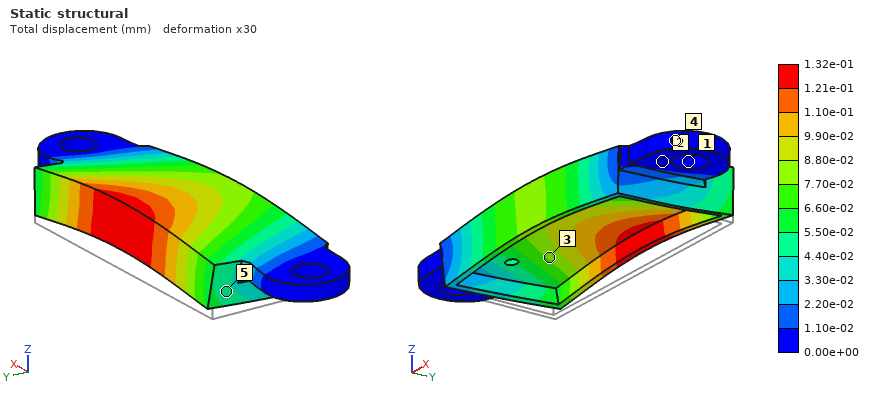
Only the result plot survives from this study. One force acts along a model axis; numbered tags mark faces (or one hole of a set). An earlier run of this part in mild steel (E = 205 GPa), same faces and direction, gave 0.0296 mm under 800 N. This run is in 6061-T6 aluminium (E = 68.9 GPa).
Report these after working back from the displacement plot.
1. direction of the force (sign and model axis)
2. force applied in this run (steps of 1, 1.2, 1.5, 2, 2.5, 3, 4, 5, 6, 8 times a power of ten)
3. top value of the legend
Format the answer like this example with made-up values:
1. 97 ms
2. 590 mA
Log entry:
1. +Z
2. 1.2 kN
3. 1.32e-01 mm
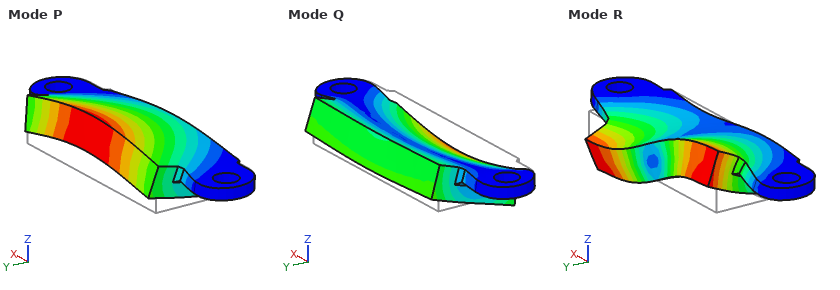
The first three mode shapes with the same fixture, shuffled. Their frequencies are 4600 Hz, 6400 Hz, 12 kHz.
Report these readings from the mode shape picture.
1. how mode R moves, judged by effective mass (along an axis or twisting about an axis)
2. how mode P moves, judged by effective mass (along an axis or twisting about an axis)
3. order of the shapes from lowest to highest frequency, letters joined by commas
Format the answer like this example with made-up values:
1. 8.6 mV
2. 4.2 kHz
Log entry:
1. twisting about Y
2. along Z
3. P, Q, R
